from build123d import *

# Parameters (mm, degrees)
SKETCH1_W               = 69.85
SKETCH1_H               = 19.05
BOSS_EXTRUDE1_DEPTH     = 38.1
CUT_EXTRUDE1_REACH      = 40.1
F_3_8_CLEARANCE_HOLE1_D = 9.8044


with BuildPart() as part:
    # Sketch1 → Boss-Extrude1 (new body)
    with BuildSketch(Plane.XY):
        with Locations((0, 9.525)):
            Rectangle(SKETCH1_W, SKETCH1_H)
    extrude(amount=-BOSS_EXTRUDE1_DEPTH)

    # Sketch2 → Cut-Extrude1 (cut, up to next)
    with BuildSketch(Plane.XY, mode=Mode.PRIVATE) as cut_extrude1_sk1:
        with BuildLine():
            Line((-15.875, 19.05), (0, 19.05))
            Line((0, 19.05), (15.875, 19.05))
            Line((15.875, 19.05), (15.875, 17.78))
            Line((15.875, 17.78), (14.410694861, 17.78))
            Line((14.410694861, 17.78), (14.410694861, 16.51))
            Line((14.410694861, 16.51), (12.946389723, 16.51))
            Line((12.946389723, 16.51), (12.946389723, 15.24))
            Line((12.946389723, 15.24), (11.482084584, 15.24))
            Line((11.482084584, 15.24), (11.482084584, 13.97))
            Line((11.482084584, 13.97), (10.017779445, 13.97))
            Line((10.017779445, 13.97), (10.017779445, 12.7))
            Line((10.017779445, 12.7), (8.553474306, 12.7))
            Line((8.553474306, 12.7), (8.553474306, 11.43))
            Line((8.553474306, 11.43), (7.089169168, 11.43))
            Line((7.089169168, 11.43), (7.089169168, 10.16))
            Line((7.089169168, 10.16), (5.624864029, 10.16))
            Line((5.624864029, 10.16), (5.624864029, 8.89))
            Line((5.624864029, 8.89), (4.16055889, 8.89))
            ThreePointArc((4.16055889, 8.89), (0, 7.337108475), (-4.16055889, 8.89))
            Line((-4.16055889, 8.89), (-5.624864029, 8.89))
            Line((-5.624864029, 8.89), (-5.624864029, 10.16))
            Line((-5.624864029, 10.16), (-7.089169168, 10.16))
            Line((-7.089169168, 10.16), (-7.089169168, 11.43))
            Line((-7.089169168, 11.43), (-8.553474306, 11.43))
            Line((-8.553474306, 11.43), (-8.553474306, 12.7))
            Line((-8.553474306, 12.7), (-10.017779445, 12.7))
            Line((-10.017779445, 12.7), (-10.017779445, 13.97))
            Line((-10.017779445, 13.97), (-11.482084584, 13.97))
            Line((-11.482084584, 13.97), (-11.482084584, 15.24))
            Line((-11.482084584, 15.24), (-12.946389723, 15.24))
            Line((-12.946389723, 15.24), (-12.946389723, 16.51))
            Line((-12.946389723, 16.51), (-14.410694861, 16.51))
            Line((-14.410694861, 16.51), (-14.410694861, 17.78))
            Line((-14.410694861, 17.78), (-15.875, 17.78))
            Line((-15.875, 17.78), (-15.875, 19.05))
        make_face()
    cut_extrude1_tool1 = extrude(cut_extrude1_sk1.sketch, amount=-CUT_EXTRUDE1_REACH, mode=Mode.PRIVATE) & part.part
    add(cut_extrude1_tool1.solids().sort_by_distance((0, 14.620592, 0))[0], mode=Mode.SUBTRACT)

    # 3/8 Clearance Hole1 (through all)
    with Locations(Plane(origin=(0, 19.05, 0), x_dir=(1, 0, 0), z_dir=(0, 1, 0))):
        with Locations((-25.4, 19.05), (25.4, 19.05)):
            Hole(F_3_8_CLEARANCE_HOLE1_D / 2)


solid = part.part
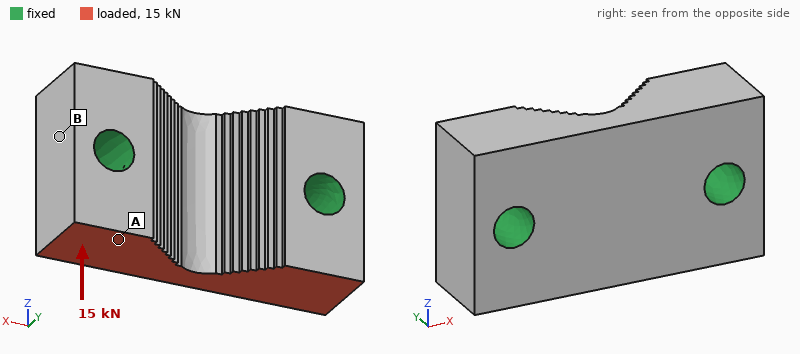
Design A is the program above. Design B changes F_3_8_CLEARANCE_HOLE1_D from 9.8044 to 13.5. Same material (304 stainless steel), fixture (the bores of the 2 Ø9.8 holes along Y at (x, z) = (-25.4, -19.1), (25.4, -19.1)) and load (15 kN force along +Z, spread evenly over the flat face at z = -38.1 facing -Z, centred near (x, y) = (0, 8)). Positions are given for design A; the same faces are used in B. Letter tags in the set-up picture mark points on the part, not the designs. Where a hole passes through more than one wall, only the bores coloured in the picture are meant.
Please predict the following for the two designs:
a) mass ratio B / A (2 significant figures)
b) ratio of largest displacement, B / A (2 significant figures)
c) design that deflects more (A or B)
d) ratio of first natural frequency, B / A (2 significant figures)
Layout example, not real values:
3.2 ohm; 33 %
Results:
0.93; 0.82; A; 1.2
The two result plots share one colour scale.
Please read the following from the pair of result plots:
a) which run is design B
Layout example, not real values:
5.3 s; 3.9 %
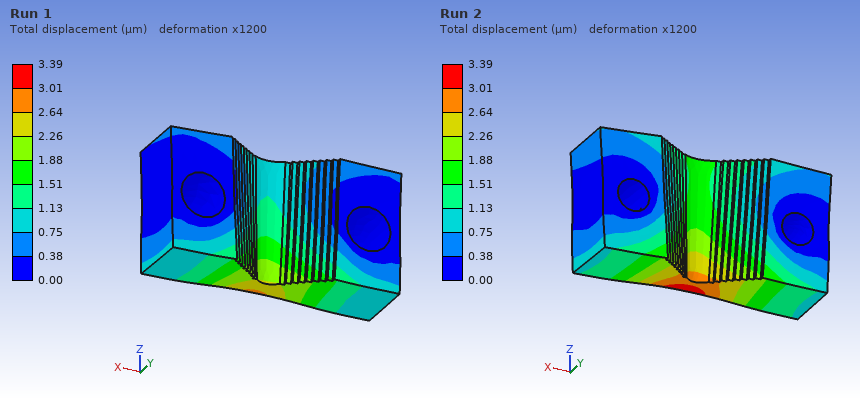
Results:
Run 1
